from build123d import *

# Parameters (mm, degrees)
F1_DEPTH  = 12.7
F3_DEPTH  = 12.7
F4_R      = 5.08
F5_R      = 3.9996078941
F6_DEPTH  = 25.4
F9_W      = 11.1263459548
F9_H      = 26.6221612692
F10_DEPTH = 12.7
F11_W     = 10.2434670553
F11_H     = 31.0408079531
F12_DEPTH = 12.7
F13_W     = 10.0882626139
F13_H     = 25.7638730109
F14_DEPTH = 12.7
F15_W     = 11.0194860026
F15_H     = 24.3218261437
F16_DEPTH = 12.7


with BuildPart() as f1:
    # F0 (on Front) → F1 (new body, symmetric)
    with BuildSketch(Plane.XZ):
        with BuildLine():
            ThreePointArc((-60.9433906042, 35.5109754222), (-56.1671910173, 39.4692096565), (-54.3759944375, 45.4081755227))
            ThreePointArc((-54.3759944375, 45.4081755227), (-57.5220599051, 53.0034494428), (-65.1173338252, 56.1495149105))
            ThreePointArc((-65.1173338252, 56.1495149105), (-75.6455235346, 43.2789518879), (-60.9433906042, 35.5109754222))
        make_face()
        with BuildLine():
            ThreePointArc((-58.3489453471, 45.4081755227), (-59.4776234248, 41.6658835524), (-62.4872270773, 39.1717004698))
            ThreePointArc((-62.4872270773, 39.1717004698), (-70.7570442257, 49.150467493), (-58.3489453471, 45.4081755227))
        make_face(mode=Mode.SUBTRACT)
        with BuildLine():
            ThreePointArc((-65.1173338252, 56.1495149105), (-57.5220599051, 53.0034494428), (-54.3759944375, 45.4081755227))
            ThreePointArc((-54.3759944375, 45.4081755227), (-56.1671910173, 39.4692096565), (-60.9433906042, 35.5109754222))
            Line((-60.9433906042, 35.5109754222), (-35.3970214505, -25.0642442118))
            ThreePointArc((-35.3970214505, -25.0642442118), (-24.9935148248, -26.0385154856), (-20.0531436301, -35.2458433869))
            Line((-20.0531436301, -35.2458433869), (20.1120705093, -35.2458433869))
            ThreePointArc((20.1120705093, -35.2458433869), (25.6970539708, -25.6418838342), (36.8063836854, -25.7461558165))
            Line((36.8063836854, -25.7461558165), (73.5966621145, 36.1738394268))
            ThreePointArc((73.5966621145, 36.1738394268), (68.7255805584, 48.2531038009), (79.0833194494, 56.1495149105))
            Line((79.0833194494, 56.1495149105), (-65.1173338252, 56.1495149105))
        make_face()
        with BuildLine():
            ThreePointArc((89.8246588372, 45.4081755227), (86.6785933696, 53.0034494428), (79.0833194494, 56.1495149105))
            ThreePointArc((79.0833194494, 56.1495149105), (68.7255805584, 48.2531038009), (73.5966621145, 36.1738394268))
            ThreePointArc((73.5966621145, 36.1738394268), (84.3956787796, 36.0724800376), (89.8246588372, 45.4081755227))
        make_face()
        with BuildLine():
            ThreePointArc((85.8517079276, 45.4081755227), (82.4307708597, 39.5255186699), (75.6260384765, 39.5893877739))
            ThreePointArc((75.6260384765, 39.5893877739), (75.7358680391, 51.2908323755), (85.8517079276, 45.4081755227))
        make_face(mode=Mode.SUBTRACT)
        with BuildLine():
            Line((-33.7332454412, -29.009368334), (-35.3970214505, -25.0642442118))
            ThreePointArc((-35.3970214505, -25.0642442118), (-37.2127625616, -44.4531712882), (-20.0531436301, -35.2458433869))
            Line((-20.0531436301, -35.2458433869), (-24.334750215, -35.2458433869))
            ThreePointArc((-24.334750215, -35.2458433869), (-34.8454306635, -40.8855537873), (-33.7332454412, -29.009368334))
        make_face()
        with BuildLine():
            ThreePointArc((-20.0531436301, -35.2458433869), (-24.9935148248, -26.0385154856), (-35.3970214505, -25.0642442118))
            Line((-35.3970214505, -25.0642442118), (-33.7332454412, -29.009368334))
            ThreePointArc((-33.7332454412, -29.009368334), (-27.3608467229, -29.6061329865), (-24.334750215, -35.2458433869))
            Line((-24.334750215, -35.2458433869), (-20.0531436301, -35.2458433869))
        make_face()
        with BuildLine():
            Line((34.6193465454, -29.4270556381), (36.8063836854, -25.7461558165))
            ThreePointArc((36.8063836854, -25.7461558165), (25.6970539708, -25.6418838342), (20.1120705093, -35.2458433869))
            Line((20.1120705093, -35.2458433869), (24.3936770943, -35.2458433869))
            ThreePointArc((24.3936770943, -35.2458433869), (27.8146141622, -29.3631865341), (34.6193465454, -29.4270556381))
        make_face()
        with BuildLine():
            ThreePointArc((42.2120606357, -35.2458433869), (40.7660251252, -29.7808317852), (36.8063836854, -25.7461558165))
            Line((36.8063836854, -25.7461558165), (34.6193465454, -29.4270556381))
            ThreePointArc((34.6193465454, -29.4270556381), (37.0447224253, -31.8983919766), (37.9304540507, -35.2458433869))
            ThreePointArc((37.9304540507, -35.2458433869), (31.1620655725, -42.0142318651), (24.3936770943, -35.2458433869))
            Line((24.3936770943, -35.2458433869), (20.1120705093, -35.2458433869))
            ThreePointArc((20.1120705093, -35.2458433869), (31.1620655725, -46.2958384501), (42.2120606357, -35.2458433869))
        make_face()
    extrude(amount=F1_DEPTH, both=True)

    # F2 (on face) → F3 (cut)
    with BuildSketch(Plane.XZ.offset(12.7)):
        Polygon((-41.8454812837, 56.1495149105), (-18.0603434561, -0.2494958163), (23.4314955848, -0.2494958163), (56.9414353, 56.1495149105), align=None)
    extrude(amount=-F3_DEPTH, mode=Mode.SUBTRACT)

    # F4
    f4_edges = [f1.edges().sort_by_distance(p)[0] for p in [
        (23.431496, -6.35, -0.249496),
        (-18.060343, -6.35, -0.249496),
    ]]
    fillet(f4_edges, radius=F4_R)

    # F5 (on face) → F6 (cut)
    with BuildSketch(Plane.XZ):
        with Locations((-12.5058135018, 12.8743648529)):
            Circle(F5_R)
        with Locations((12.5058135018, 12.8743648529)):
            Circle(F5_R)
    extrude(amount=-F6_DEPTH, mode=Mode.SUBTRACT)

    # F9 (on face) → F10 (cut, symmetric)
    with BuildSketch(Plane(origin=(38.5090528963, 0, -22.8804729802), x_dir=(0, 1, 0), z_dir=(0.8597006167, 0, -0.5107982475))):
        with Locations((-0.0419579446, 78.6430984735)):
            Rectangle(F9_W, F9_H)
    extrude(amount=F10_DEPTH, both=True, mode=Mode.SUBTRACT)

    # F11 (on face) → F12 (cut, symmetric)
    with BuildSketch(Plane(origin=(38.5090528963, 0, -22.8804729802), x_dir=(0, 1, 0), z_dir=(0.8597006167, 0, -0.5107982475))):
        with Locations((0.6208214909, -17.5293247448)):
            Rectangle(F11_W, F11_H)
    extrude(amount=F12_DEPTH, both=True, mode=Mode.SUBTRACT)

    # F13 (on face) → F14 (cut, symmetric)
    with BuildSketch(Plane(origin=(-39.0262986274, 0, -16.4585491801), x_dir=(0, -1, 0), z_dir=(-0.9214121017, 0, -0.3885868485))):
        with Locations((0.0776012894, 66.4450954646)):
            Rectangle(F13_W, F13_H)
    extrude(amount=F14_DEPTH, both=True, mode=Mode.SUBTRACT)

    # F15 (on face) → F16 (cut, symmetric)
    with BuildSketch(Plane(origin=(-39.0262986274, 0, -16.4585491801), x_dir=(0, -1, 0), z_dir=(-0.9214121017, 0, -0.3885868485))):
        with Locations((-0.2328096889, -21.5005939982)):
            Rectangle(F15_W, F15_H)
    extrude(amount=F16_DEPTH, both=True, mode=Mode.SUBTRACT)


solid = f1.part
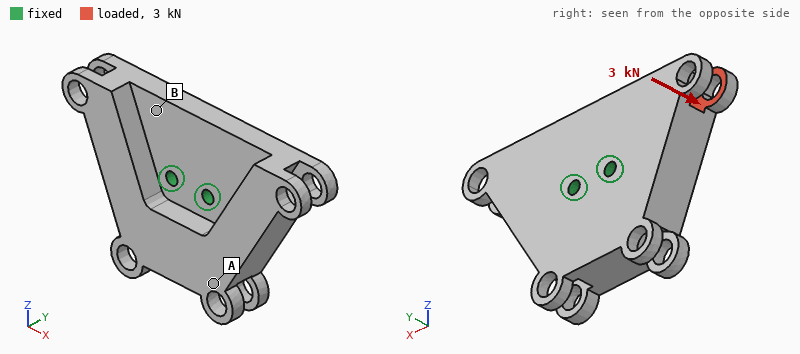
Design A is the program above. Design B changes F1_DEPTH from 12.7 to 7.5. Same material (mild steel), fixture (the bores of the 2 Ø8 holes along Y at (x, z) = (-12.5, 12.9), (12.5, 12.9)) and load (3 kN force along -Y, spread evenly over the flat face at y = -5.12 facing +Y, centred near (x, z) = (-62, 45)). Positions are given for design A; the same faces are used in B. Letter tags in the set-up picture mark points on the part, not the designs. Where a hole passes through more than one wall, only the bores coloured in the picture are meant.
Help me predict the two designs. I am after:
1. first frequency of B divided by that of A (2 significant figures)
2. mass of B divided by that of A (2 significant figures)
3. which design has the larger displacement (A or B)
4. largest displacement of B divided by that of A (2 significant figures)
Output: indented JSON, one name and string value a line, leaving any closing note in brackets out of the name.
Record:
{
  "first frequency of B divided by that of A": "0.73",
  "mass of B divided by that of A": "0.56",
  "which design has the larger displacement": "B",
  "largest displacement of B divided by that of A": "9.9"
}
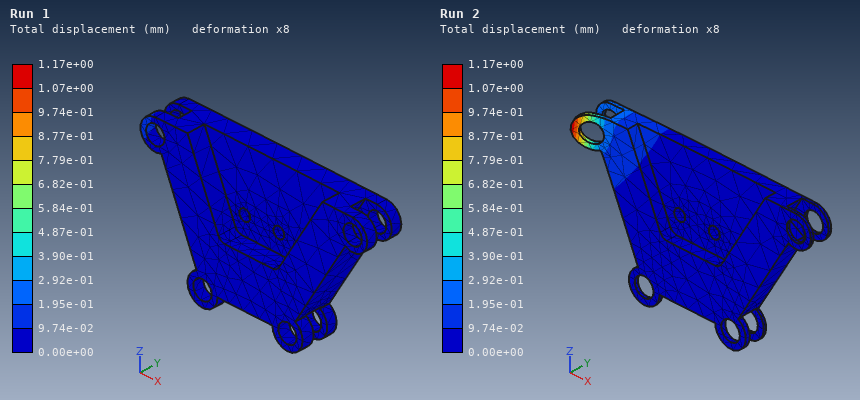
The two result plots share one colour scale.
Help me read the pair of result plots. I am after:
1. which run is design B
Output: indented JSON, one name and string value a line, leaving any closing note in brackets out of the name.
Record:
{
  "which run is design B": "Run 2"
}
